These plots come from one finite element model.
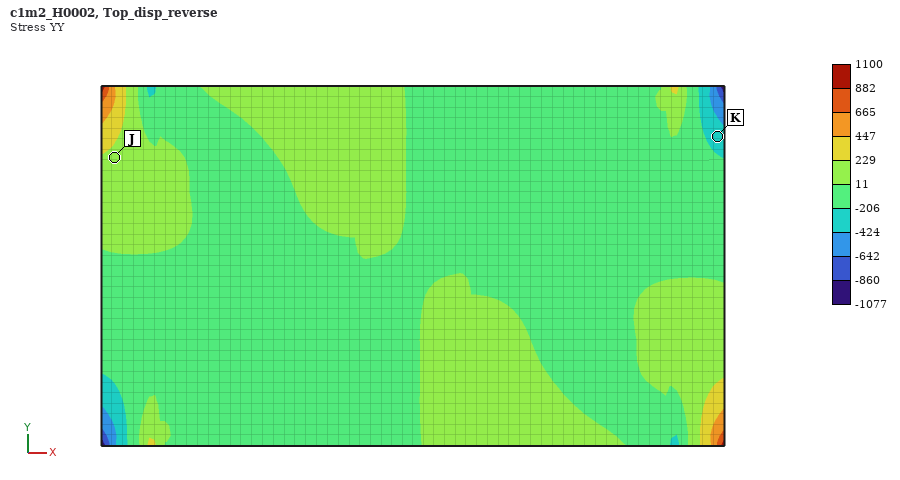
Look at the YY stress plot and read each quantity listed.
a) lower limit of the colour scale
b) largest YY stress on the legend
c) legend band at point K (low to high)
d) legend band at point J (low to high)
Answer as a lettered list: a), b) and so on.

a) -1077
b) 1100
c) -424 to -206
d) 11 to 229
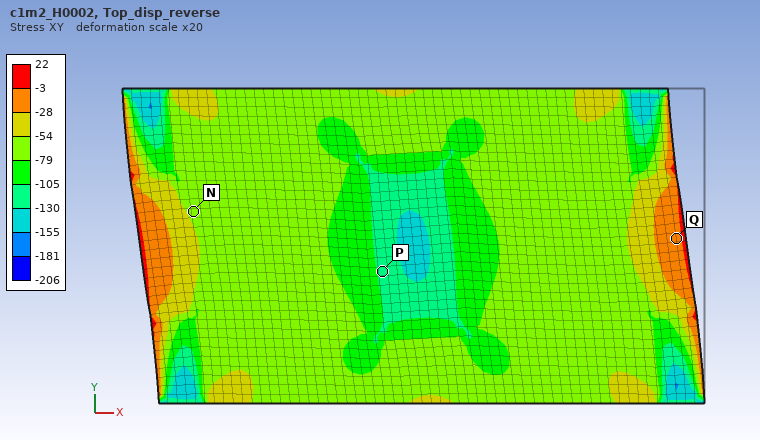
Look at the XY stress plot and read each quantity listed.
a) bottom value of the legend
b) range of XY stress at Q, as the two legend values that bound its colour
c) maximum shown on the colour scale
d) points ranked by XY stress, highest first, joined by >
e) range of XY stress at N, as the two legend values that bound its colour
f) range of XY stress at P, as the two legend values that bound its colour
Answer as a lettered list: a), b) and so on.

a) -206
b) -28 to -3
c) 22
d) Q > N > P
e) -79 to -54
f) -130 to -105
